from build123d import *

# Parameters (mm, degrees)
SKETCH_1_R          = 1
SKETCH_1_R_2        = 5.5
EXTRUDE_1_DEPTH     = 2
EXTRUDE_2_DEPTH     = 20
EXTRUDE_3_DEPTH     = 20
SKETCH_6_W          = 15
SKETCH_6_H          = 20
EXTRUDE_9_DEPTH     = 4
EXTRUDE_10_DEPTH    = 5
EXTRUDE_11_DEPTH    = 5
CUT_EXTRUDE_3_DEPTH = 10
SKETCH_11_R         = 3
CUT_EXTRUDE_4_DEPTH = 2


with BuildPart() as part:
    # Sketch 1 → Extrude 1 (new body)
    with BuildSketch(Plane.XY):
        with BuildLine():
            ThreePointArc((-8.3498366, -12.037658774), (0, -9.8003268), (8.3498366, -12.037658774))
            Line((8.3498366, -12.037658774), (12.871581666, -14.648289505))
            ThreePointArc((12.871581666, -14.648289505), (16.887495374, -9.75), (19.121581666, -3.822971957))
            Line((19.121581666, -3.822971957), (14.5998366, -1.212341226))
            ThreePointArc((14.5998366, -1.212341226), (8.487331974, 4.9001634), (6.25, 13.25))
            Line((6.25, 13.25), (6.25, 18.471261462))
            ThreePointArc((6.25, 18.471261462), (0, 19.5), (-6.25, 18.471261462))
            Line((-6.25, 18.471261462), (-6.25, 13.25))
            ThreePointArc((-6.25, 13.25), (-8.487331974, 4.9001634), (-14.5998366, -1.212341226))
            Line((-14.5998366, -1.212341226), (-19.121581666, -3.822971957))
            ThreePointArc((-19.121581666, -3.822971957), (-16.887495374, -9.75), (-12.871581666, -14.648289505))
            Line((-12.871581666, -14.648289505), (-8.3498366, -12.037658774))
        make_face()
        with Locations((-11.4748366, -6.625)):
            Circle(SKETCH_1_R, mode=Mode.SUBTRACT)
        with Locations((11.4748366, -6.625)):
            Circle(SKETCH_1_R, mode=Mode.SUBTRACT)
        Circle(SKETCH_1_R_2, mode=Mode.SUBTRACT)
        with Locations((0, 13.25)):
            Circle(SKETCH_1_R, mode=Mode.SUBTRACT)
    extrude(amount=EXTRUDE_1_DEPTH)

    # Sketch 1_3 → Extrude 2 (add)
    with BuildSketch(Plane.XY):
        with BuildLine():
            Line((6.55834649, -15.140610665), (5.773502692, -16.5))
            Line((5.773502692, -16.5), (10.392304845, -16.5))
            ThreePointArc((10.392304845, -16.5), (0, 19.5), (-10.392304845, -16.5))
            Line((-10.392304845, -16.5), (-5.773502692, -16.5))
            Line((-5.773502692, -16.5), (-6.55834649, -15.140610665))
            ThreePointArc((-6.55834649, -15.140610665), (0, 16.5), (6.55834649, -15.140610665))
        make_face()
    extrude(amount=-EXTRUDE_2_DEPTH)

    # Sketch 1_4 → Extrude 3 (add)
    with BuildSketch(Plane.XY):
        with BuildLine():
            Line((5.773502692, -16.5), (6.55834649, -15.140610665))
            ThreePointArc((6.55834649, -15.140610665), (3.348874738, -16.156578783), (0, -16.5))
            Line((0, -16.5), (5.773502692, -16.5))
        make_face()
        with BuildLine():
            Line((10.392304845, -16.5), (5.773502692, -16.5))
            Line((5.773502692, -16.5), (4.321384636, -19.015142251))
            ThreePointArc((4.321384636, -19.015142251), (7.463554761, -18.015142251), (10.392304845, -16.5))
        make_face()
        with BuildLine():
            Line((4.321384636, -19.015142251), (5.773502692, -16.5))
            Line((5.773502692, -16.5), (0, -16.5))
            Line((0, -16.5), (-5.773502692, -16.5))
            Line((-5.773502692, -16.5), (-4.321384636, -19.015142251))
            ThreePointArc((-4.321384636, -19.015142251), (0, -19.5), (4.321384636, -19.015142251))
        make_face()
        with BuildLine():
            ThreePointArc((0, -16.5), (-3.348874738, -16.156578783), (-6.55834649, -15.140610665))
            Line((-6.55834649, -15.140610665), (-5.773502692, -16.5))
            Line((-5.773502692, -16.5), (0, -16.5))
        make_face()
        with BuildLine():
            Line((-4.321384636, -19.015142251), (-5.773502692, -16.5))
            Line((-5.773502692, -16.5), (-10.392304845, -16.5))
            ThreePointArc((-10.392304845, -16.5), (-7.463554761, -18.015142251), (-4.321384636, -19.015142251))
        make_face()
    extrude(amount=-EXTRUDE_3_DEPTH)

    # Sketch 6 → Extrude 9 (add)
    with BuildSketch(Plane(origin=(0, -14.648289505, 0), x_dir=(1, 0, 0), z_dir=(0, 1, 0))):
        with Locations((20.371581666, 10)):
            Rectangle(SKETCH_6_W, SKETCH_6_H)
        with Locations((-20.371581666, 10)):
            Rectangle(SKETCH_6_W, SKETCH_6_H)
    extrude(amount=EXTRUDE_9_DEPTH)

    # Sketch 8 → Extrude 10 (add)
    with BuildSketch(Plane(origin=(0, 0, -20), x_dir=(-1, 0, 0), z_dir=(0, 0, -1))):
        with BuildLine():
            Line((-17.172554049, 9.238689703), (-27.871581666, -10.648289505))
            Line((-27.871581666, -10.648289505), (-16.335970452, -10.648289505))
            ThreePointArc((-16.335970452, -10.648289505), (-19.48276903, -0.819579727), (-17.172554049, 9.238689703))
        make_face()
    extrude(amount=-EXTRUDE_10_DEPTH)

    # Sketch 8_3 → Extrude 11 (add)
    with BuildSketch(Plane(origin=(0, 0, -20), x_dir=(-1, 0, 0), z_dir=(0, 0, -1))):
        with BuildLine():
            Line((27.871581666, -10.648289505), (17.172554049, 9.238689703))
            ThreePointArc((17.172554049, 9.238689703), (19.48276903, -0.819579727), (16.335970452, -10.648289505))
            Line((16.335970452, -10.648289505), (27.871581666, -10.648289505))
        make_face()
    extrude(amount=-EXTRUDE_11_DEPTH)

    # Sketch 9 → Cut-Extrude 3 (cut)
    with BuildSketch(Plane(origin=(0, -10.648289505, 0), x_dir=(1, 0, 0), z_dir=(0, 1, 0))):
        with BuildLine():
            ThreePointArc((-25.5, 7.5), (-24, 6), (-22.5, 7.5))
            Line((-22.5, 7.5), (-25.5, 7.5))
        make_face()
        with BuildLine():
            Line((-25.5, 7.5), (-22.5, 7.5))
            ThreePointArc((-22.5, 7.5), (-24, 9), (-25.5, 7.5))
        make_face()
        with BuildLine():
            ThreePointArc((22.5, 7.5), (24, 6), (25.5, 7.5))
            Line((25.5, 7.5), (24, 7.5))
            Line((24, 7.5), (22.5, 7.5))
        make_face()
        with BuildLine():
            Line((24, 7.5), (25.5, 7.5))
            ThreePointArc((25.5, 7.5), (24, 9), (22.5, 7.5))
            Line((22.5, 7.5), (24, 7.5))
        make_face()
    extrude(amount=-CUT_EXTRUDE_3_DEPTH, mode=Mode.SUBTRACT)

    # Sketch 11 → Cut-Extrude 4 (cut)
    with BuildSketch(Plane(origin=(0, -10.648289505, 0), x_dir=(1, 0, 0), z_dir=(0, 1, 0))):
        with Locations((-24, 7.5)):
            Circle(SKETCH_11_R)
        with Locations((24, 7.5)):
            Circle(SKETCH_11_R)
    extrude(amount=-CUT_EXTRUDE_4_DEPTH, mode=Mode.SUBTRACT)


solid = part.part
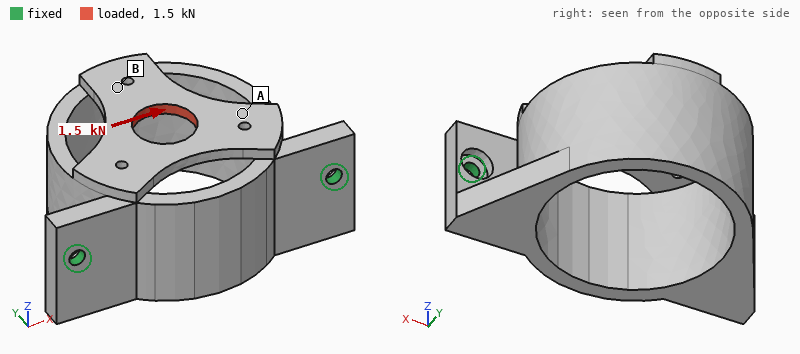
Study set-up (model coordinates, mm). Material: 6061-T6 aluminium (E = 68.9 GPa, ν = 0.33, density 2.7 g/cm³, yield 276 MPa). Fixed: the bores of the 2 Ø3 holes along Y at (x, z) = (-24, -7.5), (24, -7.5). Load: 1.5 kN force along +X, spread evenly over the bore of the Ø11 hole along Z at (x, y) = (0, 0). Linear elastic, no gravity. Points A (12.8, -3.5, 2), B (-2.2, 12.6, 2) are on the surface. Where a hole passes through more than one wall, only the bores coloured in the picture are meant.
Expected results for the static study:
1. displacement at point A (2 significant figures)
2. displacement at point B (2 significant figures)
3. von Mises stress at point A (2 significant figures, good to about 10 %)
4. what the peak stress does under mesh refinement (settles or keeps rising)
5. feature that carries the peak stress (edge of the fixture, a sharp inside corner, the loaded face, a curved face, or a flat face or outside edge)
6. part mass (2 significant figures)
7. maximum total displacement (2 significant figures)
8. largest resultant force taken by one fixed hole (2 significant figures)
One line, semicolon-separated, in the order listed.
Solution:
29 µm; 37 µm; 21 MPa; keeps rising; edge of the fixture; 29 g; 49 µm; 900 N
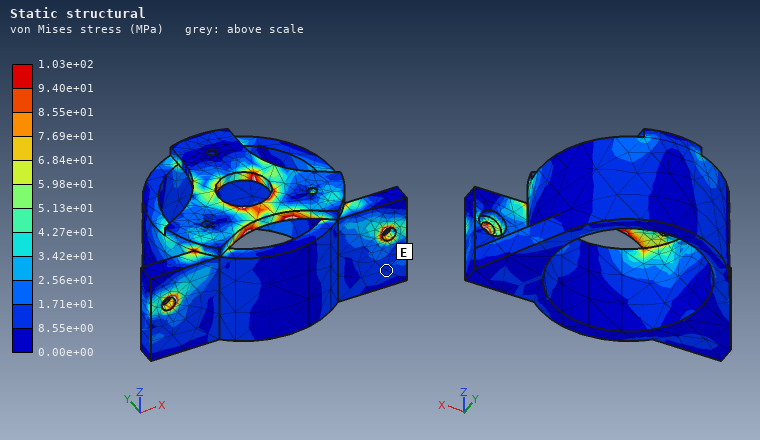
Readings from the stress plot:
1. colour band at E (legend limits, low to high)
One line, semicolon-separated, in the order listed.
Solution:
8.55e+00 to 1.71e+01 MPa
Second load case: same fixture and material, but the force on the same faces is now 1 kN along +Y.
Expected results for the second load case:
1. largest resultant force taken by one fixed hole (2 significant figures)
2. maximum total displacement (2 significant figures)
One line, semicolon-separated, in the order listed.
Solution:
570 N; 0.33 mm
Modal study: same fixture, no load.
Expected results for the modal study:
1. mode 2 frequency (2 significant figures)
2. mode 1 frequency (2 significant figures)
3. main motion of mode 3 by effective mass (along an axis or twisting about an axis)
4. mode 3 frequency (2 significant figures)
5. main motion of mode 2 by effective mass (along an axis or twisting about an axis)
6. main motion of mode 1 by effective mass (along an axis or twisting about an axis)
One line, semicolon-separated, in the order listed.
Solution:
5800 Hz; 1700 Hz; along Y; 6900 Hz; along X; along Z
